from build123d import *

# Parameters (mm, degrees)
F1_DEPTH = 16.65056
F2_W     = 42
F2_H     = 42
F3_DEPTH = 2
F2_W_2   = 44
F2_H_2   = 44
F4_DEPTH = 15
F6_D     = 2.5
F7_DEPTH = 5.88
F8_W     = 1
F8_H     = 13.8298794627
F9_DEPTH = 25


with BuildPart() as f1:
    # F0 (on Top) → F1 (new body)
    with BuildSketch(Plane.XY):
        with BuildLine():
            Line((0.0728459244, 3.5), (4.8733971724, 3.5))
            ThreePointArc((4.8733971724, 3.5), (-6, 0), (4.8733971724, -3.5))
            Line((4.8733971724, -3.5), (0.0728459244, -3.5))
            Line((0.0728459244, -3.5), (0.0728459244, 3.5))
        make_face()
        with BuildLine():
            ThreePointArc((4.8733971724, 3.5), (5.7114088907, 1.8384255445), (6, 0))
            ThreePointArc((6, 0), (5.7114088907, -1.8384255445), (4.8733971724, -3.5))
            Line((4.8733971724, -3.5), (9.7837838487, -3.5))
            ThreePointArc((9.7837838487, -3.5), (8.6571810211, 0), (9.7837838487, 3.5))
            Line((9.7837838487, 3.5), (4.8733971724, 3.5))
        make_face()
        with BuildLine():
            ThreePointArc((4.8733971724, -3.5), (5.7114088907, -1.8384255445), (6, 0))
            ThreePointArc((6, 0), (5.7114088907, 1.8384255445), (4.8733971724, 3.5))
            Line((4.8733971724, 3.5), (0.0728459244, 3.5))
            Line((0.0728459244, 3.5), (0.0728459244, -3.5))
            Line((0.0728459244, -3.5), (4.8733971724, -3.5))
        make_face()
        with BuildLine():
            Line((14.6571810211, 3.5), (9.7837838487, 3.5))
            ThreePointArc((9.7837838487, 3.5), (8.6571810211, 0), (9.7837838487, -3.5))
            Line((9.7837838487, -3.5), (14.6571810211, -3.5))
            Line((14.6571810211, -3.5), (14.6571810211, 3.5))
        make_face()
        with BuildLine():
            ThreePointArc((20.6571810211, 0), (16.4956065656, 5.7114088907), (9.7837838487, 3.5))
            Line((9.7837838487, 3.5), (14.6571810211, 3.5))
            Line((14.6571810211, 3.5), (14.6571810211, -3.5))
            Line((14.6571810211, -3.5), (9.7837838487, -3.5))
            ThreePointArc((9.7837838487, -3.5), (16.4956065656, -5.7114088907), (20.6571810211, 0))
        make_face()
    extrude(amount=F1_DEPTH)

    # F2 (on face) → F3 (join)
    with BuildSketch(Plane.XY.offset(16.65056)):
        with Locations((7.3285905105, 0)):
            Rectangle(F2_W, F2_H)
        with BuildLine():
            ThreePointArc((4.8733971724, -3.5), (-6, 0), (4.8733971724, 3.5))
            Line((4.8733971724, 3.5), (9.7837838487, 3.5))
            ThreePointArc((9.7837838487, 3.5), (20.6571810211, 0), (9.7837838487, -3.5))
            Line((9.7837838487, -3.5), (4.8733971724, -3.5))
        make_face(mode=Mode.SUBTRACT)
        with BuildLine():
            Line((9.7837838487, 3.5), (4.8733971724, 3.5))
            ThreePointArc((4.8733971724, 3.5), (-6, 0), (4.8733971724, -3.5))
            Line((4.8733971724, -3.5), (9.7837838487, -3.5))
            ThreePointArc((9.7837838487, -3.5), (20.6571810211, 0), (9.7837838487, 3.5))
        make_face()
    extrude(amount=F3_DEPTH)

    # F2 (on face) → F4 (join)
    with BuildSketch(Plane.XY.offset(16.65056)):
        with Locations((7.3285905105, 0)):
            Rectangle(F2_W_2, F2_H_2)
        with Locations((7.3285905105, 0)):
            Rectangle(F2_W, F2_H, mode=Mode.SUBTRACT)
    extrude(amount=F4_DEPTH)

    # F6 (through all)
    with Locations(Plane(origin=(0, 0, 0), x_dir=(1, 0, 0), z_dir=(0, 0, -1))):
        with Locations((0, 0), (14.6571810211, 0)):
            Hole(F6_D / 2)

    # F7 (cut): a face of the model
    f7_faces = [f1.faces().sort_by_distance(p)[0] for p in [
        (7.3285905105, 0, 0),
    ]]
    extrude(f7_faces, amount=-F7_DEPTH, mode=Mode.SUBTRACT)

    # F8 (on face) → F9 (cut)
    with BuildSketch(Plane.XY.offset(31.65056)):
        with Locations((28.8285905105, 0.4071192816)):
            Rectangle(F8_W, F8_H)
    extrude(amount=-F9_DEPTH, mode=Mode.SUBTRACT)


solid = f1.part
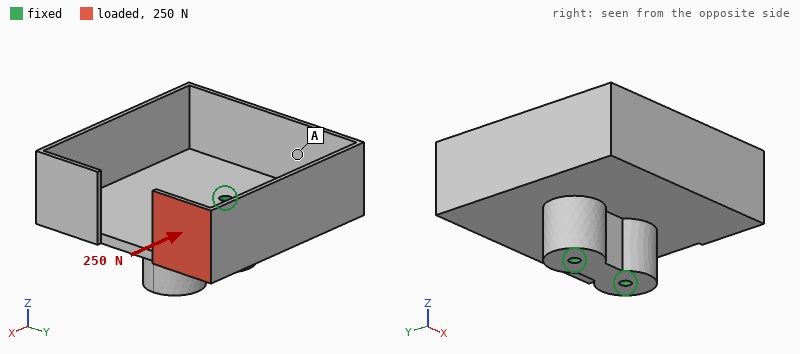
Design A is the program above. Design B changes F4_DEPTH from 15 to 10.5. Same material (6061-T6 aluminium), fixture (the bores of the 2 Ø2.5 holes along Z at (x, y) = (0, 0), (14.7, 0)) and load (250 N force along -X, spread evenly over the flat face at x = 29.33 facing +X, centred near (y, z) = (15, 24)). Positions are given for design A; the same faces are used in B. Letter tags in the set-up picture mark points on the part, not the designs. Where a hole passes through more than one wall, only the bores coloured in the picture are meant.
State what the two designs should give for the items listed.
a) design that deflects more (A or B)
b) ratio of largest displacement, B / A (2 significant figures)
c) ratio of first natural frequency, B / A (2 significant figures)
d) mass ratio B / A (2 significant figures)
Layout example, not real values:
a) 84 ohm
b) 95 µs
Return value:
a) A
b) 0.47
c) 1.2
d) 0.92
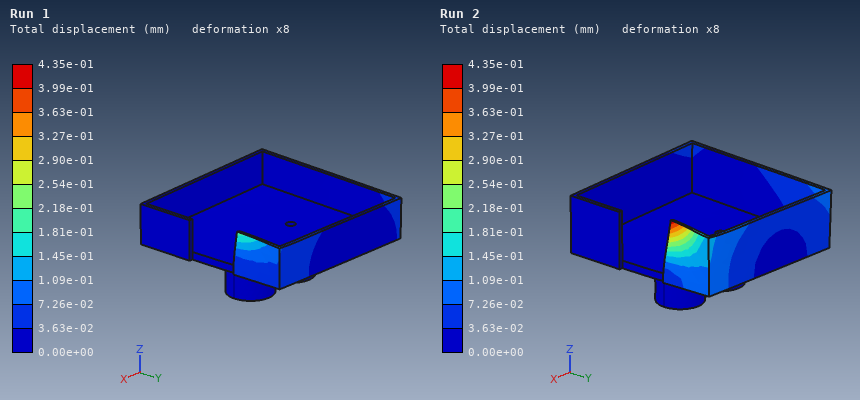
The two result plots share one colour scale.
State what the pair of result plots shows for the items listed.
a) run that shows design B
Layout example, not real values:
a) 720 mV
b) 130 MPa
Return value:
a) Run 1
